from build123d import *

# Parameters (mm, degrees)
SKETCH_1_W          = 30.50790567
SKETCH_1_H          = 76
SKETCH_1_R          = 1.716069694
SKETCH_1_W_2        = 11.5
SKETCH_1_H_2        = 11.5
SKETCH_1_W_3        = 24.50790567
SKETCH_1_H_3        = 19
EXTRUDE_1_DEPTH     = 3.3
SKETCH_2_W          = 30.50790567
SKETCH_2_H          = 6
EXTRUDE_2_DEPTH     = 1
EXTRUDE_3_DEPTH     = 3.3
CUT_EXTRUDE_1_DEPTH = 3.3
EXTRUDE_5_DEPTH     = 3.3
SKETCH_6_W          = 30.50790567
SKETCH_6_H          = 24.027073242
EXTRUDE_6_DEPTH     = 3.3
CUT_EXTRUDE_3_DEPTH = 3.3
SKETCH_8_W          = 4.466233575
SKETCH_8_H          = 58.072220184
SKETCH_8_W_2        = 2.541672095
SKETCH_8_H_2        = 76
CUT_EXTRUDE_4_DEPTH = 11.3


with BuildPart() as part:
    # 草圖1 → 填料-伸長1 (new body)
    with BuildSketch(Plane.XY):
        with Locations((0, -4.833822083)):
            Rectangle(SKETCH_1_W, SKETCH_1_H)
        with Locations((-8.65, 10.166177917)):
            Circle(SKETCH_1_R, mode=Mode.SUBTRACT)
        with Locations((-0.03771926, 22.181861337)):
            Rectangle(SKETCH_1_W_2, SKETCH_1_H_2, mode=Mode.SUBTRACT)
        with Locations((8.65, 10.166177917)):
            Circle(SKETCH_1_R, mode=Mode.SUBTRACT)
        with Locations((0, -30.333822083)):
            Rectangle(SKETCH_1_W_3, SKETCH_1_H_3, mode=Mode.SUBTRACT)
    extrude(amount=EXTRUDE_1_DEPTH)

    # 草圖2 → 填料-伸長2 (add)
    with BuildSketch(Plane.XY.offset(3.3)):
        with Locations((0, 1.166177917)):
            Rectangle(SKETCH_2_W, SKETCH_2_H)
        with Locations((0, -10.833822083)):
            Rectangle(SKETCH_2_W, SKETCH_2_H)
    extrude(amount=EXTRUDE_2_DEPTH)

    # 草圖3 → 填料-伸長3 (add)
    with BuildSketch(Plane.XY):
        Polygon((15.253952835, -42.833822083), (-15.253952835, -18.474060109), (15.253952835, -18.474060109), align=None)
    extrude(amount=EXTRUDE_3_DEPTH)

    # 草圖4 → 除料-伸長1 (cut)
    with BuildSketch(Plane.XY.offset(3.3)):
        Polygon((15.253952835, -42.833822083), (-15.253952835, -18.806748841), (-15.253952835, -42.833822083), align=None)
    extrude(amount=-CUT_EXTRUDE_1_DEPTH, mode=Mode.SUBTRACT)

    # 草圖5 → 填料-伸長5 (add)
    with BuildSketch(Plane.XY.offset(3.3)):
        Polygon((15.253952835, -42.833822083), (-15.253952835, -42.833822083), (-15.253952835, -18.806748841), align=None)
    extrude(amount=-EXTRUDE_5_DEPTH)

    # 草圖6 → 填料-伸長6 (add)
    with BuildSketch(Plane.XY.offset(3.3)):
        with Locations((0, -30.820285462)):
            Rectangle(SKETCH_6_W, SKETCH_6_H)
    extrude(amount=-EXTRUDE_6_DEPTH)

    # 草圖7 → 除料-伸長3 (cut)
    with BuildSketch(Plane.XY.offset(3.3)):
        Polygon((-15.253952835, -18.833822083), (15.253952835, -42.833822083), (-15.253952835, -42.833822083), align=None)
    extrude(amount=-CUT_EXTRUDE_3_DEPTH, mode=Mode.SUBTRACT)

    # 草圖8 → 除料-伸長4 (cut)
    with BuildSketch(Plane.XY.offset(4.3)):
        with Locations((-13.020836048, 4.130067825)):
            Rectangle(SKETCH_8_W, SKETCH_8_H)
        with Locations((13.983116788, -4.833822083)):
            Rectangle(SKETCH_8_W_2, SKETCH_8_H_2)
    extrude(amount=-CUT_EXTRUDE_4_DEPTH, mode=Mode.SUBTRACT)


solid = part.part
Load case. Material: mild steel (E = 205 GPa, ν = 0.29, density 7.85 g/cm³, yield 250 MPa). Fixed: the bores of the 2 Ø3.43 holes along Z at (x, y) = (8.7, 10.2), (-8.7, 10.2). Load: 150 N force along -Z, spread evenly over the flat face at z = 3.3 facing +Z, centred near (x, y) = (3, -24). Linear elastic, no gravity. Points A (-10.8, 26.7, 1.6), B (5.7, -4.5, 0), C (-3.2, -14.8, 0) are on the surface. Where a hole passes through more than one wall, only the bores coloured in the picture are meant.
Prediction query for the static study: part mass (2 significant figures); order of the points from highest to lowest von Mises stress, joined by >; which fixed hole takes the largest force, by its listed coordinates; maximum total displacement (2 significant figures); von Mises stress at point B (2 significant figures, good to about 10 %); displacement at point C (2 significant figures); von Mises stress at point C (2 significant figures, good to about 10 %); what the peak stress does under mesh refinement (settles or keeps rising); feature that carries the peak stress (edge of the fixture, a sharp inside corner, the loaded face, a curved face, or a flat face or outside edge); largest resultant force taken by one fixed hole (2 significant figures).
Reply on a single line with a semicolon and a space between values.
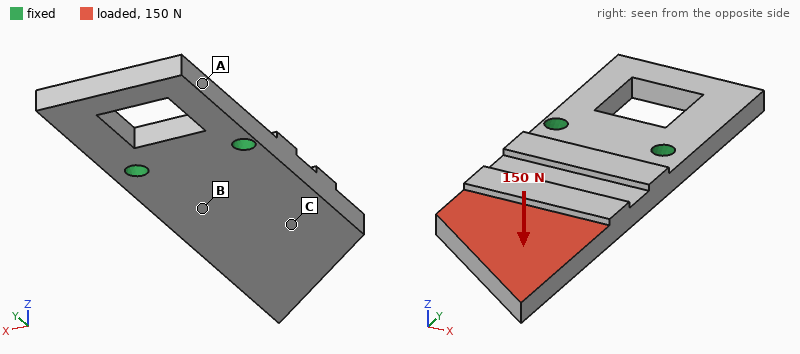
38 g; B > C > A; (8.7, 10.2); 0.20 mm; 64 MPa; 0.068 mm; 29 MPa; keeps rising; edge of the fixture; 100 N
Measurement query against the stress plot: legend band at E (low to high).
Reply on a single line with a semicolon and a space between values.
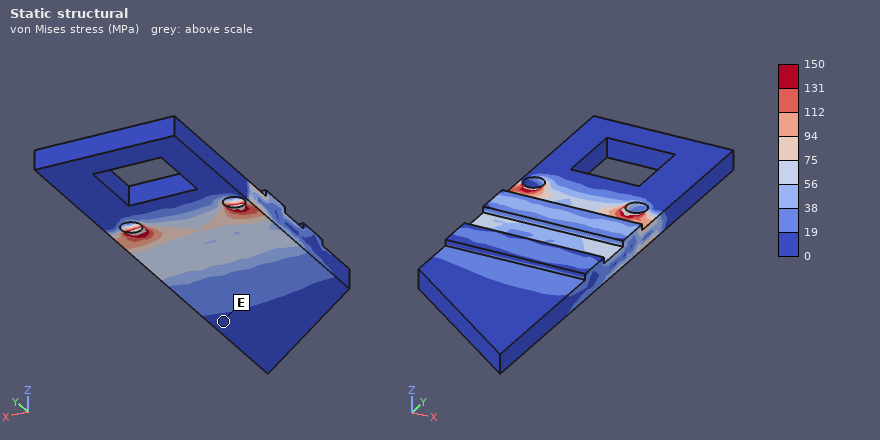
0 to 19 MPa
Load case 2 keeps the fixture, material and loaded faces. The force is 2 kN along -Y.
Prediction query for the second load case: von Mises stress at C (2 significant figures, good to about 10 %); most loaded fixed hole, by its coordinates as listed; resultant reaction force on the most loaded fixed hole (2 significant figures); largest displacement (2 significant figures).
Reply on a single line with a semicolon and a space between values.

45 MPa; (8.7, 10.2); 1.3 kN; 0.21 mm
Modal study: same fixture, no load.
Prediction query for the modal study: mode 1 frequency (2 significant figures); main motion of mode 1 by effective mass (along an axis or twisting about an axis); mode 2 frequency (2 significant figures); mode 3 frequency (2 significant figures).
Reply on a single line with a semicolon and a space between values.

1600 Hz; along Z; 4700 Hz; 6500 Hz
